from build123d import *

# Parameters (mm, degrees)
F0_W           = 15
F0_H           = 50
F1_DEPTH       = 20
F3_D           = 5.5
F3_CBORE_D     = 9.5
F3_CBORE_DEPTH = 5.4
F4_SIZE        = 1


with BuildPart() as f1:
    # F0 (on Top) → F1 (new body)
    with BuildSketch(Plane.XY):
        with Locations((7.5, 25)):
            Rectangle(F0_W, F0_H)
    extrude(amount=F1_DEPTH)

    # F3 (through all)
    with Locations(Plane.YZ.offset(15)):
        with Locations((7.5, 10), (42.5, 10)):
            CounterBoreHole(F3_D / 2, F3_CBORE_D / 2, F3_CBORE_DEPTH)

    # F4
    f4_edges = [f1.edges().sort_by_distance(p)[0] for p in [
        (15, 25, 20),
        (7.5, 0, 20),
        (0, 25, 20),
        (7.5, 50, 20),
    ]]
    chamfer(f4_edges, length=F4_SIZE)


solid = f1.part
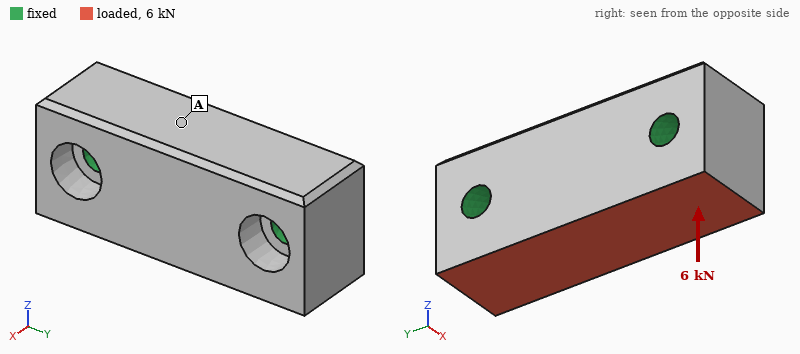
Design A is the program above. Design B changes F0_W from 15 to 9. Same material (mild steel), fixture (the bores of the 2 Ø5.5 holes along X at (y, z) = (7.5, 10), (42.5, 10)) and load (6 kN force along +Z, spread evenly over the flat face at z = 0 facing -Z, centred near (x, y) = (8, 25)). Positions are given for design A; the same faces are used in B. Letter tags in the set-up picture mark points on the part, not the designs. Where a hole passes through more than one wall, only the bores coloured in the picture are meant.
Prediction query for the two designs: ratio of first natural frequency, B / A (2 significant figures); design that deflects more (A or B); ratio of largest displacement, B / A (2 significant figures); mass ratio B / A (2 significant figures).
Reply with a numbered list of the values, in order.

1. 1.0
2. B
3. 1.2
4. 0.60
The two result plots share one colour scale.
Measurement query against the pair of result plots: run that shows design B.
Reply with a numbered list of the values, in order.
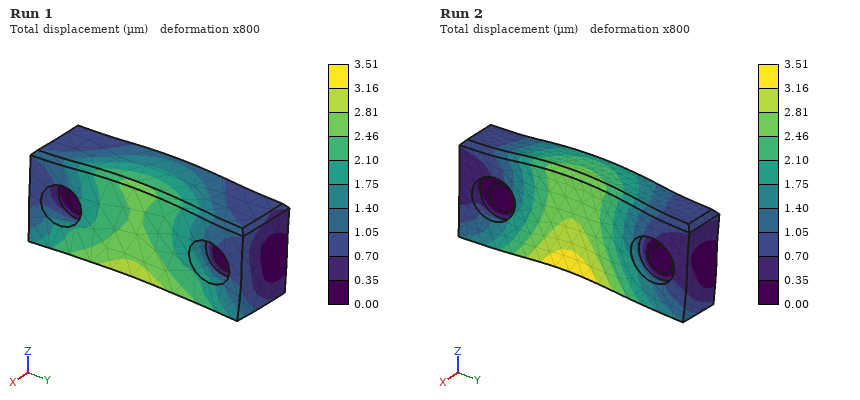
1. Run 2
